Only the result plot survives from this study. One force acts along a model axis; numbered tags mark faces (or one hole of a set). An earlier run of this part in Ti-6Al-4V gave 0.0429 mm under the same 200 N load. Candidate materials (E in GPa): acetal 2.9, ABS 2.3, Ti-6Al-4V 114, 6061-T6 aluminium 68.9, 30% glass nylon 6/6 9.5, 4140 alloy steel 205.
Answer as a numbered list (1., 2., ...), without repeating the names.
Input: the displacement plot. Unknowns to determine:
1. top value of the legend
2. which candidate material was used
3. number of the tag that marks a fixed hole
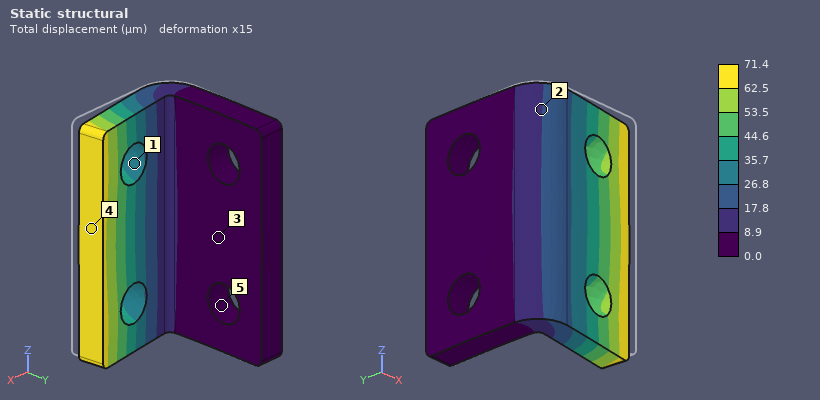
1. 71.4 µm
2. 6061-T6 aluminium
3. 5
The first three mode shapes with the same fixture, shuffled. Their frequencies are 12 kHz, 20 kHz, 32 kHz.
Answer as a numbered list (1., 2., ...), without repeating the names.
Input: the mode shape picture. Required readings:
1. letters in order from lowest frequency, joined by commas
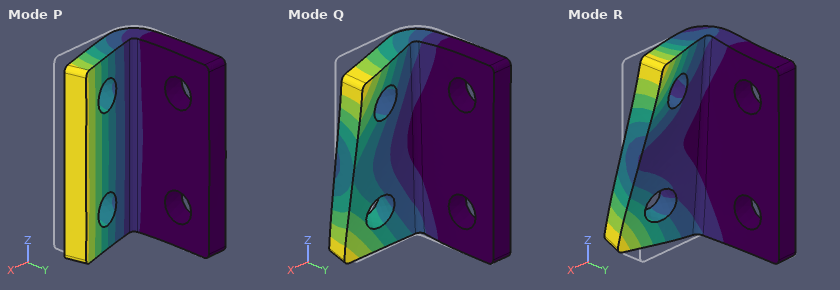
1. P, Q, R
